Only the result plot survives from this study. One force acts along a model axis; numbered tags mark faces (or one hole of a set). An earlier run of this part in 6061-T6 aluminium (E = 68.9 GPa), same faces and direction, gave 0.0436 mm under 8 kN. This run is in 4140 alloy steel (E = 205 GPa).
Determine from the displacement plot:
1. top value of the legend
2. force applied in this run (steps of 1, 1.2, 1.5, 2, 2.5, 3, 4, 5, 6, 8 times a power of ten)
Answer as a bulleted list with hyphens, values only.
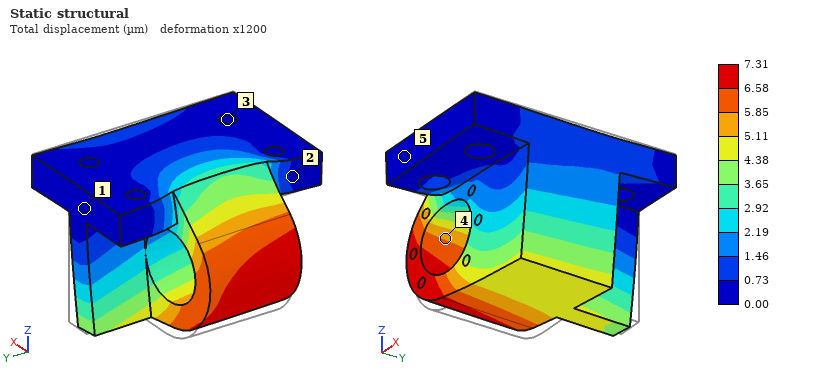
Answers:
- 7.31 µm
- 4 kN
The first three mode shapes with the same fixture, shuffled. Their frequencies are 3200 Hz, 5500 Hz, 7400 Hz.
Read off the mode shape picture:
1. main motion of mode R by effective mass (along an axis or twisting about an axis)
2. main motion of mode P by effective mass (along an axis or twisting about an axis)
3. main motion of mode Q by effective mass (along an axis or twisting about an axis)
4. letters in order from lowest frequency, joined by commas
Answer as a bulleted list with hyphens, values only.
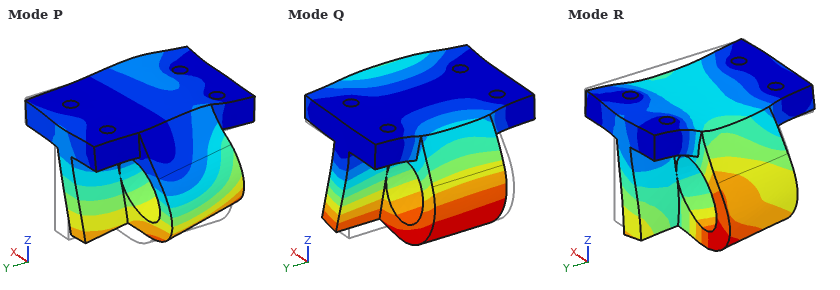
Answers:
- along Z
- along Y
- along X
- Q, P, R
